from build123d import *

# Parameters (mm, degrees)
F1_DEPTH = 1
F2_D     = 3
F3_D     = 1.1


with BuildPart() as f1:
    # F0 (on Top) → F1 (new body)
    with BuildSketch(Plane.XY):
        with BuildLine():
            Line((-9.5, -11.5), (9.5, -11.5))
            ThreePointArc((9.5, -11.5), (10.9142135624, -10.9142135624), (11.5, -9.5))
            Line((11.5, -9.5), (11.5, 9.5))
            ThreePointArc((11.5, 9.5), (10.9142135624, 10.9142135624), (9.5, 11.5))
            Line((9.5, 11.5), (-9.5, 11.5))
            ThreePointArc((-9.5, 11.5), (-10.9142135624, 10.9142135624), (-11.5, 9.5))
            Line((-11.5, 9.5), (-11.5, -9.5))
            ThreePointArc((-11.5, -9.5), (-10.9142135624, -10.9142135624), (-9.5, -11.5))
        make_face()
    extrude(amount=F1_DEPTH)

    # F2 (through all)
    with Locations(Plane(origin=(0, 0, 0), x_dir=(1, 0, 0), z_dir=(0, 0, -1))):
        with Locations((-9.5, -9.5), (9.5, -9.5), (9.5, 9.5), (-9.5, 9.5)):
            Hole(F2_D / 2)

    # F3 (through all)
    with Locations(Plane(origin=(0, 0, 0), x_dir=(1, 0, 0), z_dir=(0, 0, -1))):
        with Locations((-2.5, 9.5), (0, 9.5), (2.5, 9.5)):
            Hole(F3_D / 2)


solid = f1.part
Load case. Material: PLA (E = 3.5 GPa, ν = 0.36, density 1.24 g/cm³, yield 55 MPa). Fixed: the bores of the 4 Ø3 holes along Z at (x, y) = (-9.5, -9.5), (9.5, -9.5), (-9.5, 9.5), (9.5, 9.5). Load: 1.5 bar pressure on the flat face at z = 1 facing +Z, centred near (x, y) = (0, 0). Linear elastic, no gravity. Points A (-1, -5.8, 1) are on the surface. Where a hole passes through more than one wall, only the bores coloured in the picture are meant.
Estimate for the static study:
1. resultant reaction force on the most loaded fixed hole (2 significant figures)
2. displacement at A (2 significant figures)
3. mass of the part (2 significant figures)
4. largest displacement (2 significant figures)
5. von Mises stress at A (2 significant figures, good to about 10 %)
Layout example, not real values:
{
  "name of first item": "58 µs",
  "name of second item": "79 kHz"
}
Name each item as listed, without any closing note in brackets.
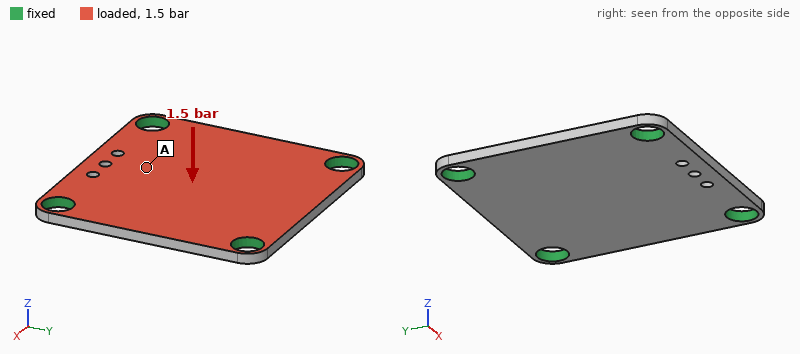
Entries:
{
  "resultant reaction force on the most loaded fixed hole": "19 N",
  "displacement at A": "0.21 mm",
  "mass of the part": "0.61 g",
  "largest displacement": "0.29 mm",
  "von Mises stress at A": "12 MPa"
}
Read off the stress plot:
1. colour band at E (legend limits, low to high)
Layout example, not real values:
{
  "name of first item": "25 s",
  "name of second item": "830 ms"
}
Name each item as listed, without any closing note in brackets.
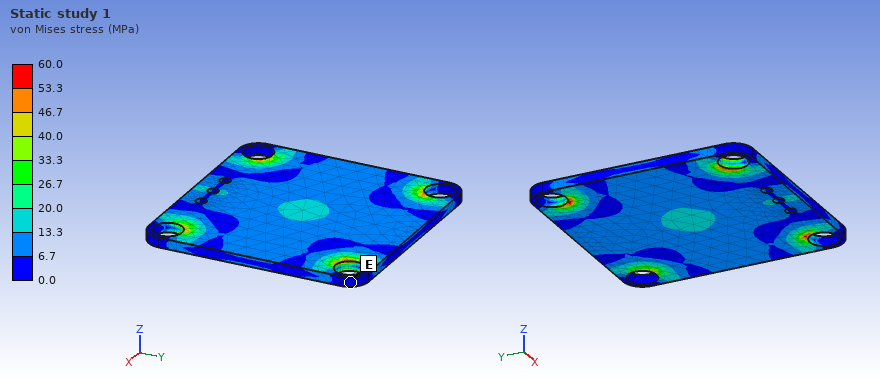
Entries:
{
  "colour band at E": "0.0 to 6.7 MPa"
}
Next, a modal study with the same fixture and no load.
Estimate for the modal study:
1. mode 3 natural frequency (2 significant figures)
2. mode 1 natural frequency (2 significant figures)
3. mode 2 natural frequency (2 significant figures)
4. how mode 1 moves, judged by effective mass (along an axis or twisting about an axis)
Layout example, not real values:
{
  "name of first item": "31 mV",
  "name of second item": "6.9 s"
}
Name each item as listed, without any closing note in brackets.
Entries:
{
  "mode 3 natural frequency": "6700 Hz",
  "mode 1 natural frequency": "4000 Hz",
  "mode 2 natural frequency": "6600 Hz",
  "how mode 1 moves, judged by effective mass": "along Z"
}
